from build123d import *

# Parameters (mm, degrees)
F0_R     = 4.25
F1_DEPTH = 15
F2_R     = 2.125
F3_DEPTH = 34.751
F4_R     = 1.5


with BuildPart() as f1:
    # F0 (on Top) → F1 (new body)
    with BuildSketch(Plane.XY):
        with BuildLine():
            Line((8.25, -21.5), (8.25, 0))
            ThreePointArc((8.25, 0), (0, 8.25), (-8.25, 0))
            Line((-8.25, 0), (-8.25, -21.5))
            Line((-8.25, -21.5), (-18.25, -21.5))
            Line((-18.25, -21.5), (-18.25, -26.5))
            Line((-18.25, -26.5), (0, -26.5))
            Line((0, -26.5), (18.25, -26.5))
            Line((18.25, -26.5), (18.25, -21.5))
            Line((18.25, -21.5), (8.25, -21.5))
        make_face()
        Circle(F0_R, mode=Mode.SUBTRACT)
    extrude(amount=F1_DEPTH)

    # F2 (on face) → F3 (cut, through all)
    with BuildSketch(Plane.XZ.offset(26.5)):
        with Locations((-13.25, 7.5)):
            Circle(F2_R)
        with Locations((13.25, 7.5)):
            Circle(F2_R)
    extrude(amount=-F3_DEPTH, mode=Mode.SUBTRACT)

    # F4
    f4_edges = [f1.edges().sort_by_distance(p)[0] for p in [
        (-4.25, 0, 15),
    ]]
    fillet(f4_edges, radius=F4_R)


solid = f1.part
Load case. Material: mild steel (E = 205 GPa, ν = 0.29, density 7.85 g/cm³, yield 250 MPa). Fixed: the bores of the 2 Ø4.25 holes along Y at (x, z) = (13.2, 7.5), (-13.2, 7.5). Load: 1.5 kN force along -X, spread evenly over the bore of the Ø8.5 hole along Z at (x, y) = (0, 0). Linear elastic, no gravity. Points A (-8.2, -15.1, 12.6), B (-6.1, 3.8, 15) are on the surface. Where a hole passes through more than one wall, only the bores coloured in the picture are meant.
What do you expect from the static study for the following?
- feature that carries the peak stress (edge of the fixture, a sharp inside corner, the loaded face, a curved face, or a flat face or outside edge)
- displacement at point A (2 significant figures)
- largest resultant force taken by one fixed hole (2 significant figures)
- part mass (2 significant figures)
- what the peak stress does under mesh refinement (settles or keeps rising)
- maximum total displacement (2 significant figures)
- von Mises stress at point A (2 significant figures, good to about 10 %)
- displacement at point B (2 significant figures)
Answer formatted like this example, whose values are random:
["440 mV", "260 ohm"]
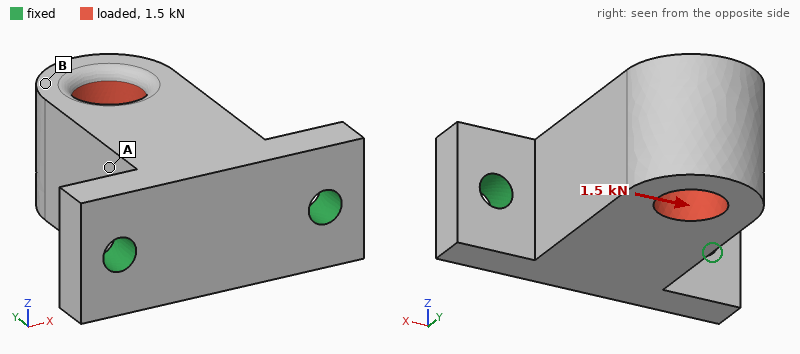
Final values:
["edge of the fixture", "6.1 µm", "1.9 kN", "68 g", "keeps rising", "23 µm", "33 MPa", "19 µm"]
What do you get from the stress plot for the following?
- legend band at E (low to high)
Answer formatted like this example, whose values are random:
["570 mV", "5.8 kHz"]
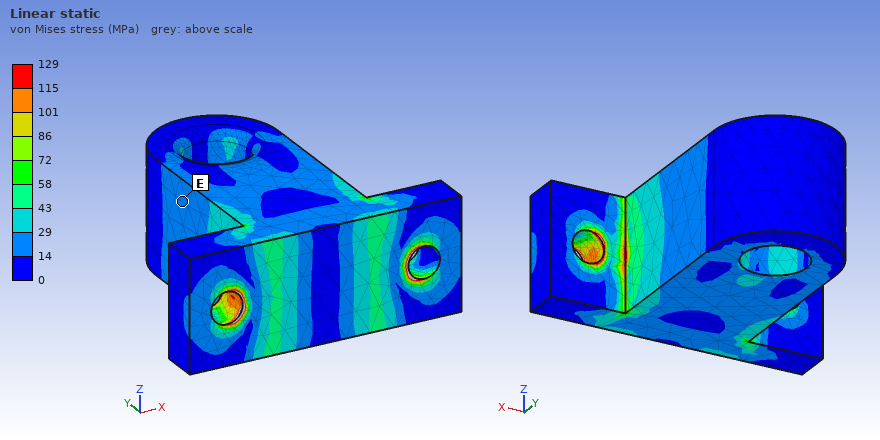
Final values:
["14 to 29 MPa"]
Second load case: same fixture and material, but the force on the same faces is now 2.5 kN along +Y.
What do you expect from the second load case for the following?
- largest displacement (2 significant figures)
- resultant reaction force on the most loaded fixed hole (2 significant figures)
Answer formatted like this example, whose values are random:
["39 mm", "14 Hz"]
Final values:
["7.7 µm", "1.3 kN"]
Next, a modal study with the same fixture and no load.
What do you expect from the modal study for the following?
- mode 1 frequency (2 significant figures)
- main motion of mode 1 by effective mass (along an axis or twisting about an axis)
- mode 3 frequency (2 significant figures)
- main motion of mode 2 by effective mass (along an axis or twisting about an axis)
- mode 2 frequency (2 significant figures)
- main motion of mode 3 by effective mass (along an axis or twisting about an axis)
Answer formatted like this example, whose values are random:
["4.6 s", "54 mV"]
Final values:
["4800 Hz", "along Z", "18 kHz", "along X", "9700 Hz", "along Y"]
